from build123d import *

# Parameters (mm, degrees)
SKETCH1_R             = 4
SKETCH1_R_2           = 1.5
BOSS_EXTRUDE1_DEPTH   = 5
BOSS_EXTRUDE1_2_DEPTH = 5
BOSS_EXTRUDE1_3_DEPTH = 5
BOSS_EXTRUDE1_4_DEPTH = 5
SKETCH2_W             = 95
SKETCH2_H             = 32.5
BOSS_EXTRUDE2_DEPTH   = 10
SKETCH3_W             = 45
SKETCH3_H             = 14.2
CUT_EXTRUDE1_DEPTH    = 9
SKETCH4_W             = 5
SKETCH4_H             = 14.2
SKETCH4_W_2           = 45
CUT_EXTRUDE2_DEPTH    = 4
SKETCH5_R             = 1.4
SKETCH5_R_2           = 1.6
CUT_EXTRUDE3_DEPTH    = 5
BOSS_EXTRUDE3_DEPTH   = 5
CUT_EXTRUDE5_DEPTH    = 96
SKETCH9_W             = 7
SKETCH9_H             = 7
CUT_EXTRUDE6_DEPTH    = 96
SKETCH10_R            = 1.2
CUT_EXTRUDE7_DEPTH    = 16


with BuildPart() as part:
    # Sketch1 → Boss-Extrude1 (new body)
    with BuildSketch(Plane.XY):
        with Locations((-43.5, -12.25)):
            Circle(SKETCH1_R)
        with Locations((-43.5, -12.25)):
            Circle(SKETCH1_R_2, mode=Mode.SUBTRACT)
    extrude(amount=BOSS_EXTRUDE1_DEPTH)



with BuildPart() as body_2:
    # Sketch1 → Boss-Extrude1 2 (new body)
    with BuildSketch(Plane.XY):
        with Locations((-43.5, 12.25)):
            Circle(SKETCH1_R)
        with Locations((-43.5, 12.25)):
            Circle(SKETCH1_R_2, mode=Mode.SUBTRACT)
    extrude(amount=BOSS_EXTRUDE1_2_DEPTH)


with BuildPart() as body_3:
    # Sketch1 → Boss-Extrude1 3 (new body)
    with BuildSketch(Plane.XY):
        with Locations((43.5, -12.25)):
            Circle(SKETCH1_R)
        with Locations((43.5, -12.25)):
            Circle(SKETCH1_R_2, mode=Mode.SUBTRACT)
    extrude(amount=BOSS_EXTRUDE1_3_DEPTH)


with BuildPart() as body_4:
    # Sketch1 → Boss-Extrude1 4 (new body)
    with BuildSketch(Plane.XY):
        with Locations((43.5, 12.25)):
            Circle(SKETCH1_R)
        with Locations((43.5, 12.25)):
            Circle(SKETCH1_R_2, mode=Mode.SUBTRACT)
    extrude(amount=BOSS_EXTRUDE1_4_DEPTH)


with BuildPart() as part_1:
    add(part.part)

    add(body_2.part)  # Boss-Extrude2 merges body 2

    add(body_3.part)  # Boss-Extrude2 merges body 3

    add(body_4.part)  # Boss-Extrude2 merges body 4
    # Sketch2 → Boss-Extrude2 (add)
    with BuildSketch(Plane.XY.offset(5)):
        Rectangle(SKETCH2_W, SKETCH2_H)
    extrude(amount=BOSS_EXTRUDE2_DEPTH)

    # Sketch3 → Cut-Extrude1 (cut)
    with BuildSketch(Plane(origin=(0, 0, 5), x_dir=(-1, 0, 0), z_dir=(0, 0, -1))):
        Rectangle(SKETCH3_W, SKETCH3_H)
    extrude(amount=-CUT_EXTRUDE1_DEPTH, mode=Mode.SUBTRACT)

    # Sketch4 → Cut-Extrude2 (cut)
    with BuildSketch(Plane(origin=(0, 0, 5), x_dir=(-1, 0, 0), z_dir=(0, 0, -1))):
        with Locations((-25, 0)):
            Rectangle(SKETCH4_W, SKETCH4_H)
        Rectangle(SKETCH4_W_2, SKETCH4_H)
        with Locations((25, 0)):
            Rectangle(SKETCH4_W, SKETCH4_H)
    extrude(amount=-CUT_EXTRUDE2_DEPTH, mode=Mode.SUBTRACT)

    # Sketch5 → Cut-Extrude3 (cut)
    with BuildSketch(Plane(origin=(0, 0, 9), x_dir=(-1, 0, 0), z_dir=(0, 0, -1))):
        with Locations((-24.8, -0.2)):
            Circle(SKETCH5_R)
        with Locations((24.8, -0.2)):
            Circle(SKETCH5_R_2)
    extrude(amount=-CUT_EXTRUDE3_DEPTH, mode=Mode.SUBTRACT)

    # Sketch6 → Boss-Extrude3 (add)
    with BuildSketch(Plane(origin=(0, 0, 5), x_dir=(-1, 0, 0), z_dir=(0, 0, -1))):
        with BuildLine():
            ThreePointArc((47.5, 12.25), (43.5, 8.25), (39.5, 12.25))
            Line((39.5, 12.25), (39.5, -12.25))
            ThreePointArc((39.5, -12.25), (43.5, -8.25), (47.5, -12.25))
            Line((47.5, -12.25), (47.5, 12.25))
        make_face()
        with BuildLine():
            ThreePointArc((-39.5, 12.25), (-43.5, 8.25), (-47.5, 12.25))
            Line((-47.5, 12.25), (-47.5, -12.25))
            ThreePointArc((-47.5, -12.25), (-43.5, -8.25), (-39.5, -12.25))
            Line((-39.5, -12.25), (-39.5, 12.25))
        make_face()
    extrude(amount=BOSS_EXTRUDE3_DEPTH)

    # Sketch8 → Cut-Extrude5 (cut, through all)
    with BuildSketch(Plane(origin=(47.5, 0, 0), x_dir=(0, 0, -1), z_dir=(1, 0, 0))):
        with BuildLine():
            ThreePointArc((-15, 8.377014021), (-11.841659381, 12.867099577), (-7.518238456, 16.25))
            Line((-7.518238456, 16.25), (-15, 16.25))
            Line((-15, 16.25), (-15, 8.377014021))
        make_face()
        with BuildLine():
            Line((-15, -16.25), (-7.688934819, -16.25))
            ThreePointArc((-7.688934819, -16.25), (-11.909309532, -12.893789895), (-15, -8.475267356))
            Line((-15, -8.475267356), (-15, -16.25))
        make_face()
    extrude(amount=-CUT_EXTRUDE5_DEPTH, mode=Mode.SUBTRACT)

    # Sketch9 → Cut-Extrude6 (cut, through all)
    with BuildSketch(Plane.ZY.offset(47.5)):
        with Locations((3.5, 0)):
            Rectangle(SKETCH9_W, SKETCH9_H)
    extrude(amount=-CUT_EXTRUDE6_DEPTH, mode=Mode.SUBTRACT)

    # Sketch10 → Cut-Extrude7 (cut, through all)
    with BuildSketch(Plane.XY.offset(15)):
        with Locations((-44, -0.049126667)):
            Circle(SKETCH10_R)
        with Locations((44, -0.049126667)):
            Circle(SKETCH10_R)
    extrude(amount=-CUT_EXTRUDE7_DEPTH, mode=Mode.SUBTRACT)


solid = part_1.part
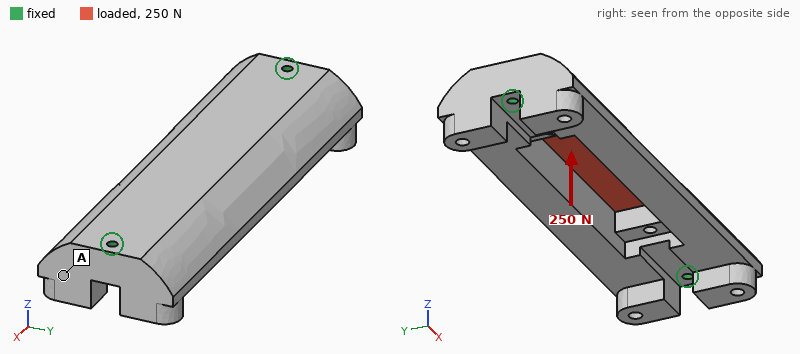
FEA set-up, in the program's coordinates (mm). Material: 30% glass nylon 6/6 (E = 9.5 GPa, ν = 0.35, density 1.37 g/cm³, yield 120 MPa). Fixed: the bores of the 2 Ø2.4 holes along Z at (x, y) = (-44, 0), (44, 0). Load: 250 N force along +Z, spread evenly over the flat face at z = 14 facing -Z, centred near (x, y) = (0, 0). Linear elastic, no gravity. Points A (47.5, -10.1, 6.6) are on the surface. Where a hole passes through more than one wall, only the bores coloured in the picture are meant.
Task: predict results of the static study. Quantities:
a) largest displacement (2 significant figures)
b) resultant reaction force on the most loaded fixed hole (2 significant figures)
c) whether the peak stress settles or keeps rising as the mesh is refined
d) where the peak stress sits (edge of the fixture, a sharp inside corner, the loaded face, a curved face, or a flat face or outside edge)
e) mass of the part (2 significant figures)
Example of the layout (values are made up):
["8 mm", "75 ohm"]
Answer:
["0.14 mm", "150 N", "keeps rising", "edge of the fixture", "29 g"]
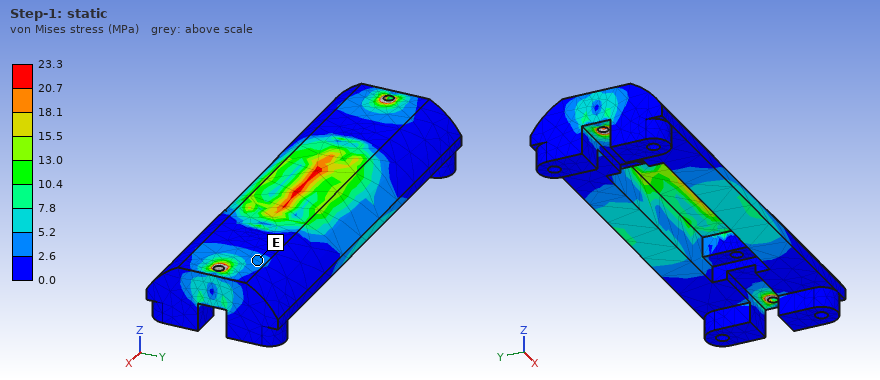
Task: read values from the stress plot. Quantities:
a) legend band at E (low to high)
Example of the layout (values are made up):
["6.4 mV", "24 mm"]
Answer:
["2.6 to 5.2 MPa"]
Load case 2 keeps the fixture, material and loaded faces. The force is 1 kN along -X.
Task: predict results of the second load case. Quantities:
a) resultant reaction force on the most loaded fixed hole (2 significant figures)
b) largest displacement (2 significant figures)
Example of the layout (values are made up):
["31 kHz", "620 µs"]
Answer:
["500 N", "30 µm"]
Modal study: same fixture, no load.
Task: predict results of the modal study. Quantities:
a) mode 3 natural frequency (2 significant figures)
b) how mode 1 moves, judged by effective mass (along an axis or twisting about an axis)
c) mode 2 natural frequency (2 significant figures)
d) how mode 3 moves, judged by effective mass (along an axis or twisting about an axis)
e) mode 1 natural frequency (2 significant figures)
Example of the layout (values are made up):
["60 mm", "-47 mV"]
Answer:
["4600 Hz", "along Z", "3100 Hz", "along Y", "2500 Hz"]
